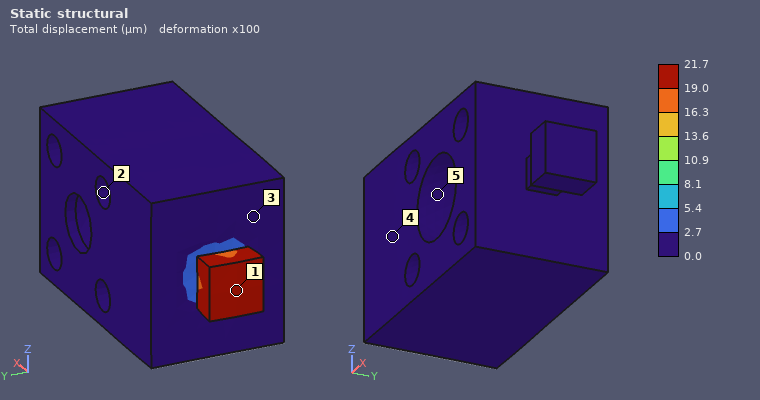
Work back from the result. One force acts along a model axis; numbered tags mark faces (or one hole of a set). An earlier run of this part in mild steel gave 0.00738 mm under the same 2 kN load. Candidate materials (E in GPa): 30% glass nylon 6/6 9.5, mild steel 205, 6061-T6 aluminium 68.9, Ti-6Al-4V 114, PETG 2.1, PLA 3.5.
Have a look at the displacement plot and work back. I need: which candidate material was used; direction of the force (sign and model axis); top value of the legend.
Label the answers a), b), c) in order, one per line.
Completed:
a) 6061-T6 aluminium
b) +X
c) 21.7 µm
